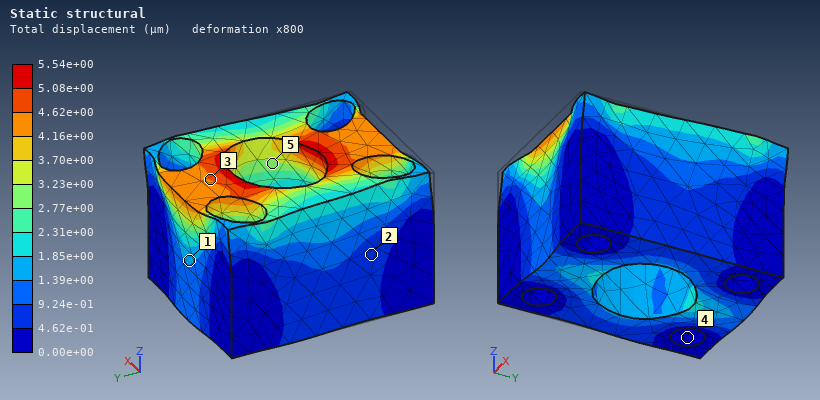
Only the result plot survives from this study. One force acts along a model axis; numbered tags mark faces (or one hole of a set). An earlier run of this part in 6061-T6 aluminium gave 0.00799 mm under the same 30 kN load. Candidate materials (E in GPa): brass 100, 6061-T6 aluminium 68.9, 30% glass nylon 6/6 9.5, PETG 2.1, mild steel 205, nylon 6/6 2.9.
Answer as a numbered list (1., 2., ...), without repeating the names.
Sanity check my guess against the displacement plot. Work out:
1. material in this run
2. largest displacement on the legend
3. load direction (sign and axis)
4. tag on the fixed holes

1. brass
2. 5.54e+00 µm
3. +Y
4. 4
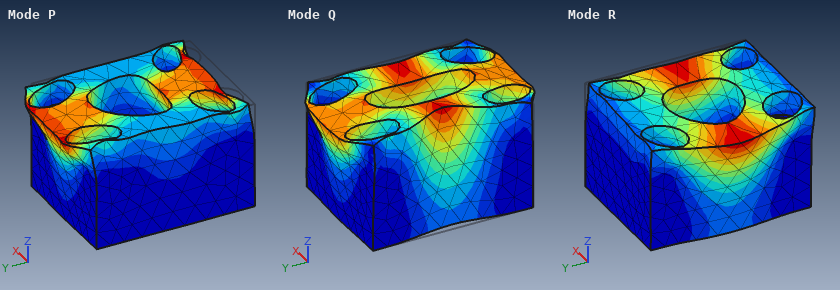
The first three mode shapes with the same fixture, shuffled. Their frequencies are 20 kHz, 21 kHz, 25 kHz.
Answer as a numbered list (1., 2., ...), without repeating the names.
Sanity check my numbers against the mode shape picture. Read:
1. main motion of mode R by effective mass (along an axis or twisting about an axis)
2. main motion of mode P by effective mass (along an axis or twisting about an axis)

1. along X
2. along Y
